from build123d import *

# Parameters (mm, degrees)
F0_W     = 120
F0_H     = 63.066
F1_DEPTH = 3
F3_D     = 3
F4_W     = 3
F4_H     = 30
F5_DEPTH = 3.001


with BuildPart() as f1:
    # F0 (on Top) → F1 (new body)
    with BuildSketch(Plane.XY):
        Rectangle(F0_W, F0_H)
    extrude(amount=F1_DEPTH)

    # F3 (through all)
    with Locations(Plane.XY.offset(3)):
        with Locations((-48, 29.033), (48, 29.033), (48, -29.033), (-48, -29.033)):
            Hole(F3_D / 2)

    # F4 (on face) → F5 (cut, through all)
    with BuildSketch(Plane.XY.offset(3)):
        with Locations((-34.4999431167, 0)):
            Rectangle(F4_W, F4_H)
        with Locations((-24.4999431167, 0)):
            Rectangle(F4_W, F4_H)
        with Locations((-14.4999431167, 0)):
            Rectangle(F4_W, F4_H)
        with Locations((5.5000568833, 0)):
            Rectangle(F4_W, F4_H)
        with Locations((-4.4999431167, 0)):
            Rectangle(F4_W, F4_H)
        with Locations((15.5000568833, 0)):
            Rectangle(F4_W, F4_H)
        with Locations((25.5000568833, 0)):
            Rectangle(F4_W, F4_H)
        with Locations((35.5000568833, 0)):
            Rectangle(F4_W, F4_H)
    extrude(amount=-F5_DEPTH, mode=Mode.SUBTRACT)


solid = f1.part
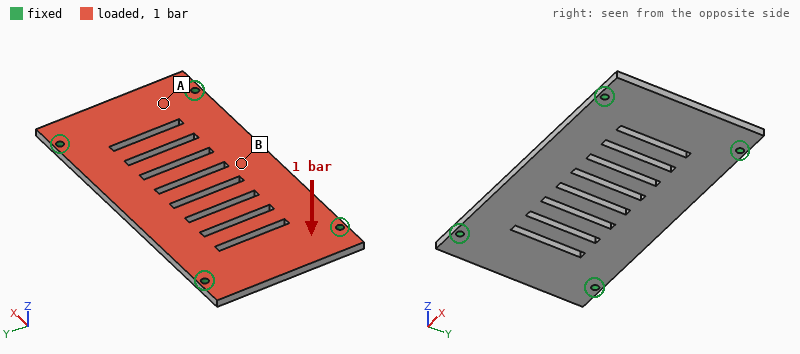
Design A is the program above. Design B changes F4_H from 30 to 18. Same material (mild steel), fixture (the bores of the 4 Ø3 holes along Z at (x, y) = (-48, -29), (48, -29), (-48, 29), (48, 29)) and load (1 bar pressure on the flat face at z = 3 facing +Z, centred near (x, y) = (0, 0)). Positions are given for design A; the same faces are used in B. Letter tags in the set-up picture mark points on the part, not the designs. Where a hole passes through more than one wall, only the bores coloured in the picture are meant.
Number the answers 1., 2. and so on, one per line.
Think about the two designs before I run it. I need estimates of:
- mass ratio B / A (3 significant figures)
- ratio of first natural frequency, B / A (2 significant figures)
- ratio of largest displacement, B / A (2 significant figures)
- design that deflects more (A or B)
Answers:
1. 1.04
2. 1.0
3. 0.90
4. A
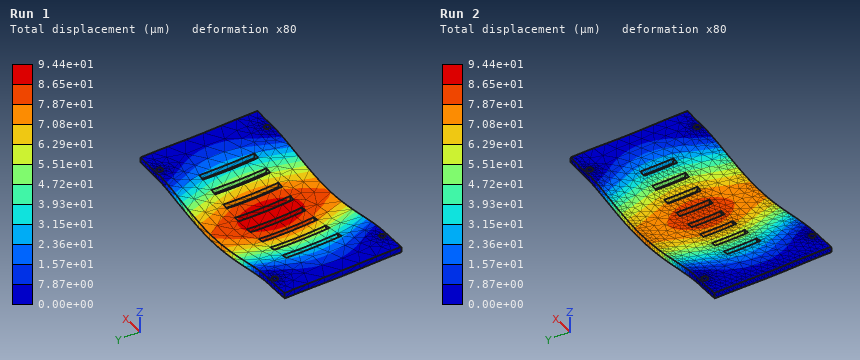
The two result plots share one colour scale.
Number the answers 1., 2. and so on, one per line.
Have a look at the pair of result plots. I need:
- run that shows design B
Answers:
1. Run 2
